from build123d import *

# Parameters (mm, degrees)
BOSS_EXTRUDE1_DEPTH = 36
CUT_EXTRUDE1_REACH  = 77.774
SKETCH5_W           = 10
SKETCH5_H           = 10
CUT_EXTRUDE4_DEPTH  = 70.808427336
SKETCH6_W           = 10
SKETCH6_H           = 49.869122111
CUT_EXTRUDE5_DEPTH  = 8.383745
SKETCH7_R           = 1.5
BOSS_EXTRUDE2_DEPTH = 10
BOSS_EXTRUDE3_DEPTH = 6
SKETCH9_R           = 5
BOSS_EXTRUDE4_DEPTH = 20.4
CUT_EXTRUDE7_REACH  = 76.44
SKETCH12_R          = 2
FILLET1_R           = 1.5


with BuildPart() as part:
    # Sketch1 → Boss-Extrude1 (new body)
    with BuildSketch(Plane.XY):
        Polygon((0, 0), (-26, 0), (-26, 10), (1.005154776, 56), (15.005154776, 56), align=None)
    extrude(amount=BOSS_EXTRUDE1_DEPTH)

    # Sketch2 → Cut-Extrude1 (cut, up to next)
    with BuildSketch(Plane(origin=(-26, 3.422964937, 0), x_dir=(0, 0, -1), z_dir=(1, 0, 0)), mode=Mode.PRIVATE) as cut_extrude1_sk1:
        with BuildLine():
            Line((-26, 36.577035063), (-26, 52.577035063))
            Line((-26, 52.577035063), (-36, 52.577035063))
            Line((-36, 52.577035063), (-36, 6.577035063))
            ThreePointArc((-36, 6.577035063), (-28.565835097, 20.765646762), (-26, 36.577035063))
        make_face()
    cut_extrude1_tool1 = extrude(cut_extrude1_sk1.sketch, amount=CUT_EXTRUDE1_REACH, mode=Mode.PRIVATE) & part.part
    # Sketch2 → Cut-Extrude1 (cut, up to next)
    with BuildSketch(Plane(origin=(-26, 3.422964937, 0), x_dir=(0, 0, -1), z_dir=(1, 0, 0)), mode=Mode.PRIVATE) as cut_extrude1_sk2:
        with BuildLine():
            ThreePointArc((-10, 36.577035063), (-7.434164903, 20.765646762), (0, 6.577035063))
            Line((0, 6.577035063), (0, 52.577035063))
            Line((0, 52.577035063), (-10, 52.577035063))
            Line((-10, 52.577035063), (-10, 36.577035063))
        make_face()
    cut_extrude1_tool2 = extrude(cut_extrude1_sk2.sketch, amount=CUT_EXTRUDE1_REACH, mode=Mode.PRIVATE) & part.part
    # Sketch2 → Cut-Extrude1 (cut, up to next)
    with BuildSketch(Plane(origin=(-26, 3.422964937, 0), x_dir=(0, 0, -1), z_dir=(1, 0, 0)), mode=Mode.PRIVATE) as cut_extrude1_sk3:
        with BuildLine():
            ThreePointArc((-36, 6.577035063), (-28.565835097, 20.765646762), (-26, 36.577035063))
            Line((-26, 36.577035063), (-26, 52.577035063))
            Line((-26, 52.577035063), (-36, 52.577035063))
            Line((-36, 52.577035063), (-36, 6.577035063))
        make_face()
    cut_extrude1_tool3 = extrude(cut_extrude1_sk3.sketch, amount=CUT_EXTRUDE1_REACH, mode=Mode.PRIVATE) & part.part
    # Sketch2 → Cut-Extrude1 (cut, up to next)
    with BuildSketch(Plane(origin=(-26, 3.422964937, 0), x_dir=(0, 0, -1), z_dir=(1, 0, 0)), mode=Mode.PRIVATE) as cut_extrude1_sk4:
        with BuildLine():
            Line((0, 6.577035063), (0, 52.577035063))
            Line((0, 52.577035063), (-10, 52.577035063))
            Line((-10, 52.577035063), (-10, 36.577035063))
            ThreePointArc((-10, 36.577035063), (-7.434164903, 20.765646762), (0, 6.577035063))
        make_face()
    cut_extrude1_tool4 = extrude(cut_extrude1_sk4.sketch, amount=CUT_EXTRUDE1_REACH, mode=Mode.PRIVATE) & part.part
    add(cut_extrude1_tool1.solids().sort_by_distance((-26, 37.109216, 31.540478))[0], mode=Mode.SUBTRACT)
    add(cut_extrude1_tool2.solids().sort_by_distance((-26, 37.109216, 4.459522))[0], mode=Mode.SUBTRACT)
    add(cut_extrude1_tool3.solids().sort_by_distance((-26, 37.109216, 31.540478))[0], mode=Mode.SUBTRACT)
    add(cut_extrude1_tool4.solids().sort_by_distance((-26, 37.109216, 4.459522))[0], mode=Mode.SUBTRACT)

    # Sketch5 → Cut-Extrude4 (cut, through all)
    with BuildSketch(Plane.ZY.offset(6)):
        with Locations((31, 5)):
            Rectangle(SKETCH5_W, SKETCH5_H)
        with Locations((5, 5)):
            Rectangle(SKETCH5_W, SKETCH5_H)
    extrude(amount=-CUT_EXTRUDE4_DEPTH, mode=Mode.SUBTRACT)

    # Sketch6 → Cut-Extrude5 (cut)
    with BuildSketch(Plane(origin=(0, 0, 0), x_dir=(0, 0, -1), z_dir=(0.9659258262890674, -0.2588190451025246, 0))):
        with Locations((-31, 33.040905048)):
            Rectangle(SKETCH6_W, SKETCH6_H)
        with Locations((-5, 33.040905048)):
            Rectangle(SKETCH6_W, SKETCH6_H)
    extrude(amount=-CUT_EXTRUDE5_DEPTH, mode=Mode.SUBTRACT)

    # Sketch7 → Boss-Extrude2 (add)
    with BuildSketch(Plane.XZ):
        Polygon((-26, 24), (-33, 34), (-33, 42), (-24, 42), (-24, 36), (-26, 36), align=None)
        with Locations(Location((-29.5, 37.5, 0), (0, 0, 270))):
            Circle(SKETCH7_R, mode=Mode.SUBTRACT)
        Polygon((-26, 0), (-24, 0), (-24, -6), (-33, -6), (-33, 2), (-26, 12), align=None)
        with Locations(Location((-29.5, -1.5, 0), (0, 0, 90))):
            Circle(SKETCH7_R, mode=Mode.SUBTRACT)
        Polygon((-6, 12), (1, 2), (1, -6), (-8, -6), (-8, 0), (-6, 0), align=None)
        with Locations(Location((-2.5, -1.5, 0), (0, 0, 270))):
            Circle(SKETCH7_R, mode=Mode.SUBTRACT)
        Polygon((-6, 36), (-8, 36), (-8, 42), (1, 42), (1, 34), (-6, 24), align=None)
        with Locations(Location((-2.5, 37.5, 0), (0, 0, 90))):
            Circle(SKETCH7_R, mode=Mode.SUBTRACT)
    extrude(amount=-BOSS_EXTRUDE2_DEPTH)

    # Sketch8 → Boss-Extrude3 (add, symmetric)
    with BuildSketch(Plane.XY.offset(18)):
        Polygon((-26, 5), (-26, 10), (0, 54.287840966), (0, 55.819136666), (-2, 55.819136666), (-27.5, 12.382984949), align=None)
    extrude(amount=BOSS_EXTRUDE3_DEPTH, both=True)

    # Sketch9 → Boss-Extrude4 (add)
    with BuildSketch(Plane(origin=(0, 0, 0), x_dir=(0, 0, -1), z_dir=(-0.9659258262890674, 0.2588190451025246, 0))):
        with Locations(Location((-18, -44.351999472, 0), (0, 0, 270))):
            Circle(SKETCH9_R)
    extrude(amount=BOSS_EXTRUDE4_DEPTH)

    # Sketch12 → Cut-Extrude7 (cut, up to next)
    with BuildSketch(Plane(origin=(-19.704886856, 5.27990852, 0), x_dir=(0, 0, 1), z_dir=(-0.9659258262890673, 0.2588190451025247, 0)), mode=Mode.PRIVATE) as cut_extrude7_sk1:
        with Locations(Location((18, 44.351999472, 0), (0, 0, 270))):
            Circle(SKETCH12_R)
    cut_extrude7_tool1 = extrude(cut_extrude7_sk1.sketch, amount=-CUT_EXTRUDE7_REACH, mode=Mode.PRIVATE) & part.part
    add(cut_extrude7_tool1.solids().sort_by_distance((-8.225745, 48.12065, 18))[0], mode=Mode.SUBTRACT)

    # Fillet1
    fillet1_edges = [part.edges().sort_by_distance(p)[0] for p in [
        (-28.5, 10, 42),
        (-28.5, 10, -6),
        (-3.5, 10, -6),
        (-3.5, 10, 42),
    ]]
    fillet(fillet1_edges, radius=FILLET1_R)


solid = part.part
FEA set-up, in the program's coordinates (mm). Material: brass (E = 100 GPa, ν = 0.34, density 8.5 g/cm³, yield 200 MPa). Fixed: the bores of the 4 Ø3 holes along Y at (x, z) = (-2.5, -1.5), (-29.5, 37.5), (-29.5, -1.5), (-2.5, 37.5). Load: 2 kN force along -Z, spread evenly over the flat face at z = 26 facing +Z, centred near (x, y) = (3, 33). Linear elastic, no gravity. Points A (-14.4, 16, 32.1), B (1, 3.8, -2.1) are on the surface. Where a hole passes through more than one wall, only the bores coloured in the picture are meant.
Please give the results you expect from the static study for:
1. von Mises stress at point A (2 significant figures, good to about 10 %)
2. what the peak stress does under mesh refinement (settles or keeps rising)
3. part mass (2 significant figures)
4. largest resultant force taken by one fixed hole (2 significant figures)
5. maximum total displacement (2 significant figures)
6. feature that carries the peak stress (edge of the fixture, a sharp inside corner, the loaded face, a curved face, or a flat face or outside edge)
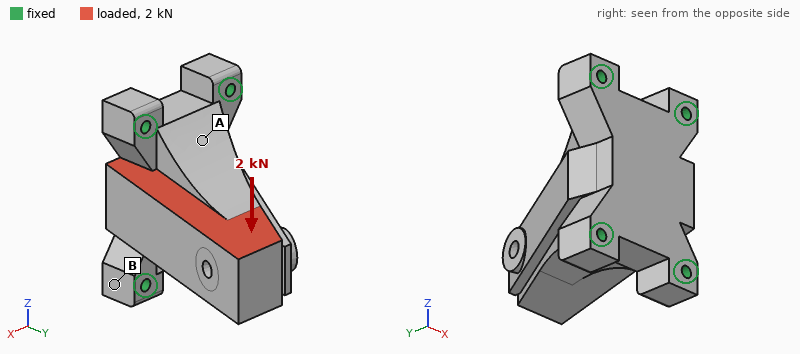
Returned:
18 MPa
keeps rising
280 g
1.1 kN
43 µm
edge of the fixture
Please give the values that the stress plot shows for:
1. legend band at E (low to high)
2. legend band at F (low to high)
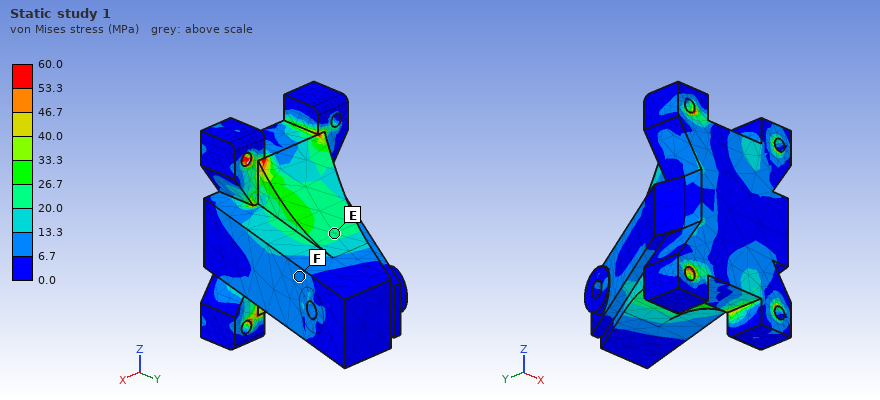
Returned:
20.0 to 26.7 MPa
6.7 to 13.3 MPa
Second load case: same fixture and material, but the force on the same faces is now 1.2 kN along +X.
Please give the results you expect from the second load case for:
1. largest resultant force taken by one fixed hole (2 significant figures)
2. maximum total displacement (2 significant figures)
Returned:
850 N
34 µm
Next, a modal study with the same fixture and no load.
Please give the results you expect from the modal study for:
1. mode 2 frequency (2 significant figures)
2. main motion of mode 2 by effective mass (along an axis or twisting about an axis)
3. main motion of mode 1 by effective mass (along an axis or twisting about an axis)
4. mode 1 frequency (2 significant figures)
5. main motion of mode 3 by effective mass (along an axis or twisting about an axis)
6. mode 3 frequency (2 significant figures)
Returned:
4400 Hz
along Z
along X
3400 Hz
along Y
9100 Hz
